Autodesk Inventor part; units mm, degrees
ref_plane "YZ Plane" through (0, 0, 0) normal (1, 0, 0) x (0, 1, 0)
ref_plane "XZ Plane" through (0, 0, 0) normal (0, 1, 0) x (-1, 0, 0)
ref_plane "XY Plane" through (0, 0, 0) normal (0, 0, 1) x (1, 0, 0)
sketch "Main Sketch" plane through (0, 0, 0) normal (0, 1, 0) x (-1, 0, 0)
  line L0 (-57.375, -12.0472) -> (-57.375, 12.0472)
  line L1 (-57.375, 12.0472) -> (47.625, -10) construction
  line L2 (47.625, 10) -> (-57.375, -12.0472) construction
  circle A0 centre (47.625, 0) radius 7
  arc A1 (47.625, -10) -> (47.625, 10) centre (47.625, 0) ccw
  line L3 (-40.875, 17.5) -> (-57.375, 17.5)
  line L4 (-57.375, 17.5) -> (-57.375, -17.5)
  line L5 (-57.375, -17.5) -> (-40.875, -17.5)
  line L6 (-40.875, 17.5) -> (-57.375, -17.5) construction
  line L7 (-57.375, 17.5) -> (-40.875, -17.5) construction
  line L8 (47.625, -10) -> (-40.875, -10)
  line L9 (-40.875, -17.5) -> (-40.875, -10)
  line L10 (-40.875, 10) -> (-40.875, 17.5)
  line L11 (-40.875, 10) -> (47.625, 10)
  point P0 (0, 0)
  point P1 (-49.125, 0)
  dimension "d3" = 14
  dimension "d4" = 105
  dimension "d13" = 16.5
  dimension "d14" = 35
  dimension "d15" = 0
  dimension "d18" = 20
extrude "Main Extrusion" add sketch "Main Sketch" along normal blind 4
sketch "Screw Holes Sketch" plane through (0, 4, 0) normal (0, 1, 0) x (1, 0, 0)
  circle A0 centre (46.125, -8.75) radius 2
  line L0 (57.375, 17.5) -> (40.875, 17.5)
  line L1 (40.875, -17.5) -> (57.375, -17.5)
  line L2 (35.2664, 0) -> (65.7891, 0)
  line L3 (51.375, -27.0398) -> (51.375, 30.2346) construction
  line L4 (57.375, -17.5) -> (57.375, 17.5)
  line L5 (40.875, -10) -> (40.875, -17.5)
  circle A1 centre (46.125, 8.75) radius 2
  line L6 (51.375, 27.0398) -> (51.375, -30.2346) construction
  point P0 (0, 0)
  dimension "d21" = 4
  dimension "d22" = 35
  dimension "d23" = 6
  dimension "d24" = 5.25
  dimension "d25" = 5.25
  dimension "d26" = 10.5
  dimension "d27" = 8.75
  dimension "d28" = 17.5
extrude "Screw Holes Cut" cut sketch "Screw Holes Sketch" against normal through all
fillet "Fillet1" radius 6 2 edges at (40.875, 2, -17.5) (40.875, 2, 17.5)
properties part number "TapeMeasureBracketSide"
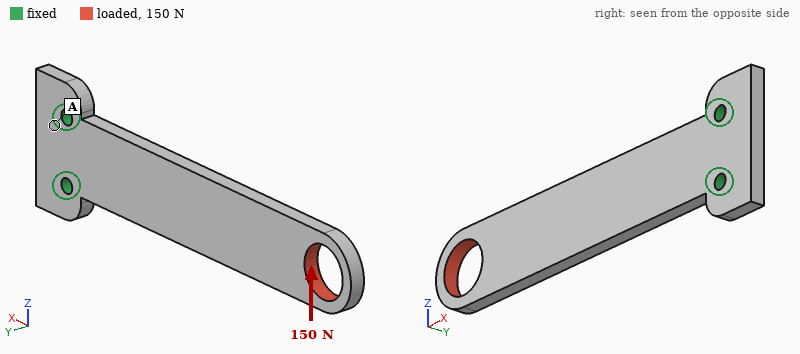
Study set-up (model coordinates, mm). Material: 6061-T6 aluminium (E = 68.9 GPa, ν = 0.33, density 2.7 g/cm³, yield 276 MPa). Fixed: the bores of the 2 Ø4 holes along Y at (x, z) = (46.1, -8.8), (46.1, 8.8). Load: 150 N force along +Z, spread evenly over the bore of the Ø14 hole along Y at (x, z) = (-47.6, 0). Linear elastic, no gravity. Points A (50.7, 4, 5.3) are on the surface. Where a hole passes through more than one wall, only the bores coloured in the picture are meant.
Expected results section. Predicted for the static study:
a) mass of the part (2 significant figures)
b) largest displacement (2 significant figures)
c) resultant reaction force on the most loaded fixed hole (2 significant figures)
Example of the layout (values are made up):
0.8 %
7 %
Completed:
25 g
0.26 mm
790 N
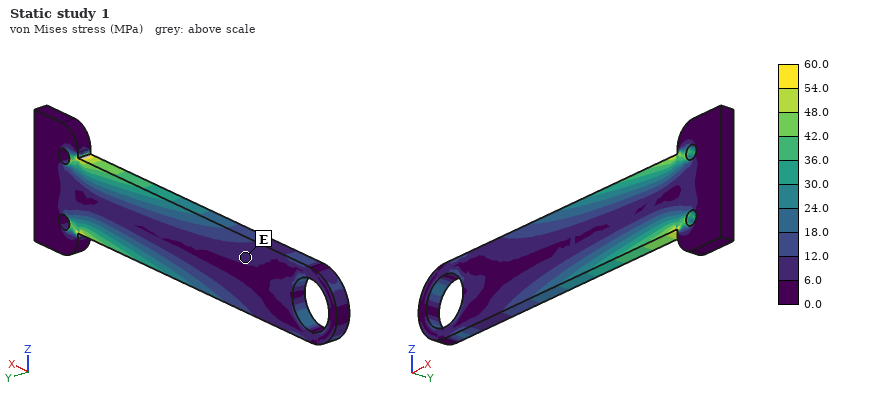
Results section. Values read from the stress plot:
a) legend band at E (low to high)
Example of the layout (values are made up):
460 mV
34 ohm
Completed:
6.0 to 12.0 MPa
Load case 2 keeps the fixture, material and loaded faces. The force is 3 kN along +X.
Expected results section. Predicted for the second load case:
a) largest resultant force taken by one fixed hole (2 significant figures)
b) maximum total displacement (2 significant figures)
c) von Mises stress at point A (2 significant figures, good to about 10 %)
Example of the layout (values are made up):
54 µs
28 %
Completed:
1.5 kN
93 µm
15 MPa
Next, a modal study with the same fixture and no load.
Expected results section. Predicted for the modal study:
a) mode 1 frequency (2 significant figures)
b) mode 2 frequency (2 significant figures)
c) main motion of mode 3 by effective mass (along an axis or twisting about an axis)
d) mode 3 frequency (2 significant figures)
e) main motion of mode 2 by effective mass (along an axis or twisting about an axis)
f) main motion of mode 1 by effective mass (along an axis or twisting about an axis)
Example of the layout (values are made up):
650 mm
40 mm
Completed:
370 Hz
1800 Hz
along Y
2200 Hz
along Z
along Y
